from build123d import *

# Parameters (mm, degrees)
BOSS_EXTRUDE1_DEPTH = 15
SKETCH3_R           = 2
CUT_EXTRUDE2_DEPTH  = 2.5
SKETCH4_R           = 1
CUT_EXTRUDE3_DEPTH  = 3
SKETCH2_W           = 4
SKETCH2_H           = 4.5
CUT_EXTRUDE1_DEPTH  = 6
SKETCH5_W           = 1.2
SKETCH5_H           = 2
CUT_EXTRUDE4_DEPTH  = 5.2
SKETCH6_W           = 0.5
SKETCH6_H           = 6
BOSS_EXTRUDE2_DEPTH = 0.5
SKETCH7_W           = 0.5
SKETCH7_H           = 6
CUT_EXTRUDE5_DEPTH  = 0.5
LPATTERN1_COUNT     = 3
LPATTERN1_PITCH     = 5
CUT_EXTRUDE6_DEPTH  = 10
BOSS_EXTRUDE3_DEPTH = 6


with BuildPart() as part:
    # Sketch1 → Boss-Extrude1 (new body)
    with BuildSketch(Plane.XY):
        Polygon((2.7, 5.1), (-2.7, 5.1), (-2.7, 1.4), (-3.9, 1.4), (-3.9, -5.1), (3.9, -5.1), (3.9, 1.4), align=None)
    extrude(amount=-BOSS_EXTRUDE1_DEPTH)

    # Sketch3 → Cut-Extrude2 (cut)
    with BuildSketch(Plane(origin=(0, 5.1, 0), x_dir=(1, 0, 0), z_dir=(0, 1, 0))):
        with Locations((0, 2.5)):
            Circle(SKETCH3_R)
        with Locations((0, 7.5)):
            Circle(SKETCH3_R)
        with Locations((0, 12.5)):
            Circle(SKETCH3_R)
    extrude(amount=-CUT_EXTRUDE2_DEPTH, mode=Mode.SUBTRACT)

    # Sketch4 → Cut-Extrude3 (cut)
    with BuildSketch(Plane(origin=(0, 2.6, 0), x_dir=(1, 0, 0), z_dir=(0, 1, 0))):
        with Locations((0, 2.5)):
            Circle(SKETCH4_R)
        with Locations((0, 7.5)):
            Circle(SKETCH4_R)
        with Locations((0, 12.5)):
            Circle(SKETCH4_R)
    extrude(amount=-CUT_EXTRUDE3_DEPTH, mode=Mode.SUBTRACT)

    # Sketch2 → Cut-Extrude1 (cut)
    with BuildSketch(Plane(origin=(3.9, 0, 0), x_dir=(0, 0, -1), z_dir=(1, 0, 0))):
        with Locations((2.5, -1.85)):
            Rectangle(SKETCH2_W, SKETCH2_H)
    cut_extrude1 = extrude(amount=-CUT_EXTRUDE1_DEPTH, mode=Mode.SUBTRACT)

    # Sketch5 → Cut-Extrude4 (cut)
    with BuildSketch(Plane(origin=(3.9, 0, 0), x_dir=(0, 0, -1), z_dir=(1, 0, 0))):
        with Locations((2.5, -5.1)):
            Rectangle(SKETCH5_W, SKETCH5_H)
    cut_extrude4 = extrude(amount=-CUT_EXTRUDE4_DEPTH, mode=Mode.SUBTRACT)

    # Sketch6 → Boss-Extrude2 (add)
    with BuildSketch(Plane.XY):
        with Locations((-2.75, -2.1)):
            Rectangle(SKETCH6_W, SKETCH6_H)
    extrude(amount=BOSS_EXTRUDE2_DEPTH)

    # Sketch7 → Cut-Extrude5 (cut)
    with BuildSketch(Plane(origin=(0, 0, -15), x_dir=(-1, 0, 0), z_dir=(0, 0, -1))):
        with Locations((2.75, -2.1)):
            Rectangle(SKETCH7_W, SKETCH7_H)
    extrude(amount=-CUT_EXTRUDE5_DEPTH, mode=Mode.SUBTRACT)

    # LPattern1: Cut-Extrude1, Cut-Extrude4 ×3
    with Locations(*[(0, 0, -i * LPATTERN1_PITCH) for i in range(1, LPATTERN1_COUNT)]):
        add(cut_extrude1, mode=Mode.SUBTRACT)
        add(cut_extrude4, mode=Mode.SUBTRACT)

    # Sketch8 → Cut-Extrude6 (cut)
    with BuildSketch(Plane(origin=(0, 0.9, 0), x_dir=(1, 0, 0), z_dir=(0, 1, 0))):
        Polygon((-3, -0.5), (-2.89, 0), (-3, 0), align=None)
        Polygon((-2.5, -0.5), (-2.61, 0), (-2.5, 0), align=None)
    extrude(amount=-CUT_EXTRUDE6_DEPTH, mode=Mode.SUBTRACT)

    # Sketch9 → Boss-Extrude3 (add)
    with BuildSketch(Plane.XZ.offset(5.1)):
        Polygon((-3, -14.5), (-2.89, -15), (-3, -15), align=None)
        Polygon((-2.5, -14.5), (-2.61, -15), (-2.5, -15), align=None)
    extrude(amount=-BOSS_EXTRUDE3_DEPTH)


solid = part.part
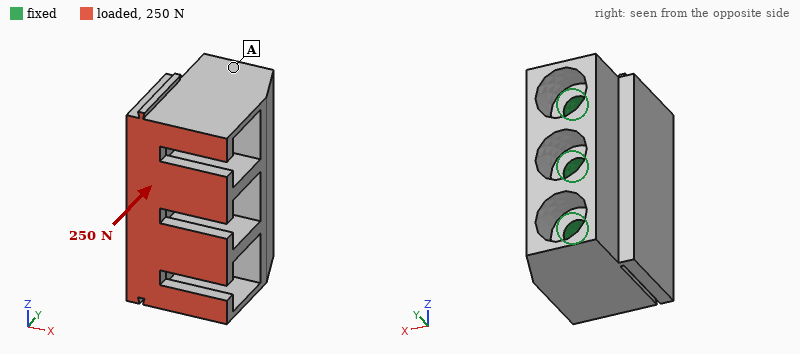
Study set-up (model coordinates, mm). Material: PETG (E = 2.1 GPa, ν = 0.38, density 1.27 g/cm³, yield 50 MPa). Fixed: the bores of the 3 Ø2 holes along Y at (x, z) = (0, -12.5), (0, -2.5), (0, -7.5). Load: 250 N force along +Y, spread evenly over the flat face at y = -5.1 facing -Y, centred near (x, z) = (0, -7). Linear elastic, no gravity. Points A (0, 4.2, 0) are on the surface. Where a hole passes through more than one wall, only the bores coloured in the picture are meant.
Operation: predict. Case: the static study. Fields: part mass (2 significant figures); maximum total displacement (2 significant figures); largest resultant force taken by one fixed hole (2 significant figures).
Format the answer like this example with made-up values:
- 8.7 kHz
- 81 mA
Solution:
- 0.81 g
- 0.21 mm
- 86 N
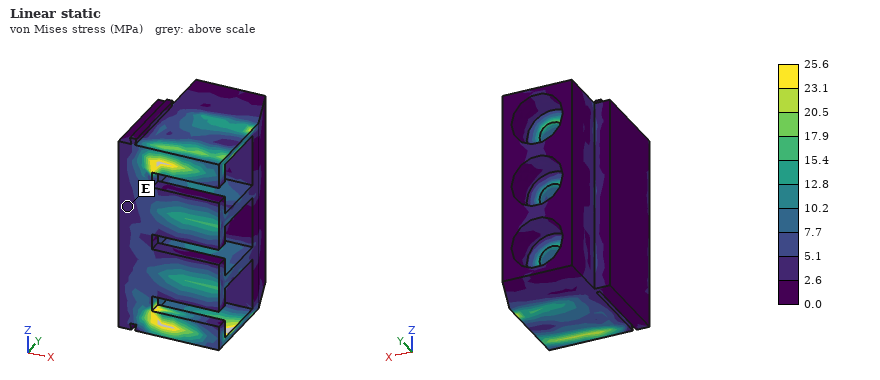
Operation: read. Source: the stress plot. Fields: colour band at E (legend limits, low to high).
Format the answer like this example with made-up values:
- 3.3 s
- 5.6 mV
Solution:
- 2.6 to 5.1 MPa
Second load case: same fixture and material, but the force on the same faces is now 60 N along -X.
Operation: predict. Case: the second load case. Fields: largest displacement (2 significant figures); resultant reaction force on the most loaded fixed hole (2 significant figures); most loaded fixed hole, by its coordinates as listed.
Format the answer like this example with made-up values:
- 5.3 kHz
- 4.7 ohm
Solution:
- 0.11 mm
- 23 N
- (0, -7.5)
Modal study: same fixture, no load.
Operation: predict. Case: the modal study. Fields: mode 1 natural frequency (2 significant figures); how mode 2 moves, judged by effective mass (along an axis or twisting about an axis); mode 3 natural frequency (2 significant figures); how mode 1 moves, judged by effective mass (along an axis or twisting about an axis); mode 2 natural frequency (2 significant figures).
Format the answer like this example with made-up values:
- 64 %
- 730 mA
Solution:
- 8000 Hz
- along X
- 9500 Hz
- along Z
- 8800 Hz
